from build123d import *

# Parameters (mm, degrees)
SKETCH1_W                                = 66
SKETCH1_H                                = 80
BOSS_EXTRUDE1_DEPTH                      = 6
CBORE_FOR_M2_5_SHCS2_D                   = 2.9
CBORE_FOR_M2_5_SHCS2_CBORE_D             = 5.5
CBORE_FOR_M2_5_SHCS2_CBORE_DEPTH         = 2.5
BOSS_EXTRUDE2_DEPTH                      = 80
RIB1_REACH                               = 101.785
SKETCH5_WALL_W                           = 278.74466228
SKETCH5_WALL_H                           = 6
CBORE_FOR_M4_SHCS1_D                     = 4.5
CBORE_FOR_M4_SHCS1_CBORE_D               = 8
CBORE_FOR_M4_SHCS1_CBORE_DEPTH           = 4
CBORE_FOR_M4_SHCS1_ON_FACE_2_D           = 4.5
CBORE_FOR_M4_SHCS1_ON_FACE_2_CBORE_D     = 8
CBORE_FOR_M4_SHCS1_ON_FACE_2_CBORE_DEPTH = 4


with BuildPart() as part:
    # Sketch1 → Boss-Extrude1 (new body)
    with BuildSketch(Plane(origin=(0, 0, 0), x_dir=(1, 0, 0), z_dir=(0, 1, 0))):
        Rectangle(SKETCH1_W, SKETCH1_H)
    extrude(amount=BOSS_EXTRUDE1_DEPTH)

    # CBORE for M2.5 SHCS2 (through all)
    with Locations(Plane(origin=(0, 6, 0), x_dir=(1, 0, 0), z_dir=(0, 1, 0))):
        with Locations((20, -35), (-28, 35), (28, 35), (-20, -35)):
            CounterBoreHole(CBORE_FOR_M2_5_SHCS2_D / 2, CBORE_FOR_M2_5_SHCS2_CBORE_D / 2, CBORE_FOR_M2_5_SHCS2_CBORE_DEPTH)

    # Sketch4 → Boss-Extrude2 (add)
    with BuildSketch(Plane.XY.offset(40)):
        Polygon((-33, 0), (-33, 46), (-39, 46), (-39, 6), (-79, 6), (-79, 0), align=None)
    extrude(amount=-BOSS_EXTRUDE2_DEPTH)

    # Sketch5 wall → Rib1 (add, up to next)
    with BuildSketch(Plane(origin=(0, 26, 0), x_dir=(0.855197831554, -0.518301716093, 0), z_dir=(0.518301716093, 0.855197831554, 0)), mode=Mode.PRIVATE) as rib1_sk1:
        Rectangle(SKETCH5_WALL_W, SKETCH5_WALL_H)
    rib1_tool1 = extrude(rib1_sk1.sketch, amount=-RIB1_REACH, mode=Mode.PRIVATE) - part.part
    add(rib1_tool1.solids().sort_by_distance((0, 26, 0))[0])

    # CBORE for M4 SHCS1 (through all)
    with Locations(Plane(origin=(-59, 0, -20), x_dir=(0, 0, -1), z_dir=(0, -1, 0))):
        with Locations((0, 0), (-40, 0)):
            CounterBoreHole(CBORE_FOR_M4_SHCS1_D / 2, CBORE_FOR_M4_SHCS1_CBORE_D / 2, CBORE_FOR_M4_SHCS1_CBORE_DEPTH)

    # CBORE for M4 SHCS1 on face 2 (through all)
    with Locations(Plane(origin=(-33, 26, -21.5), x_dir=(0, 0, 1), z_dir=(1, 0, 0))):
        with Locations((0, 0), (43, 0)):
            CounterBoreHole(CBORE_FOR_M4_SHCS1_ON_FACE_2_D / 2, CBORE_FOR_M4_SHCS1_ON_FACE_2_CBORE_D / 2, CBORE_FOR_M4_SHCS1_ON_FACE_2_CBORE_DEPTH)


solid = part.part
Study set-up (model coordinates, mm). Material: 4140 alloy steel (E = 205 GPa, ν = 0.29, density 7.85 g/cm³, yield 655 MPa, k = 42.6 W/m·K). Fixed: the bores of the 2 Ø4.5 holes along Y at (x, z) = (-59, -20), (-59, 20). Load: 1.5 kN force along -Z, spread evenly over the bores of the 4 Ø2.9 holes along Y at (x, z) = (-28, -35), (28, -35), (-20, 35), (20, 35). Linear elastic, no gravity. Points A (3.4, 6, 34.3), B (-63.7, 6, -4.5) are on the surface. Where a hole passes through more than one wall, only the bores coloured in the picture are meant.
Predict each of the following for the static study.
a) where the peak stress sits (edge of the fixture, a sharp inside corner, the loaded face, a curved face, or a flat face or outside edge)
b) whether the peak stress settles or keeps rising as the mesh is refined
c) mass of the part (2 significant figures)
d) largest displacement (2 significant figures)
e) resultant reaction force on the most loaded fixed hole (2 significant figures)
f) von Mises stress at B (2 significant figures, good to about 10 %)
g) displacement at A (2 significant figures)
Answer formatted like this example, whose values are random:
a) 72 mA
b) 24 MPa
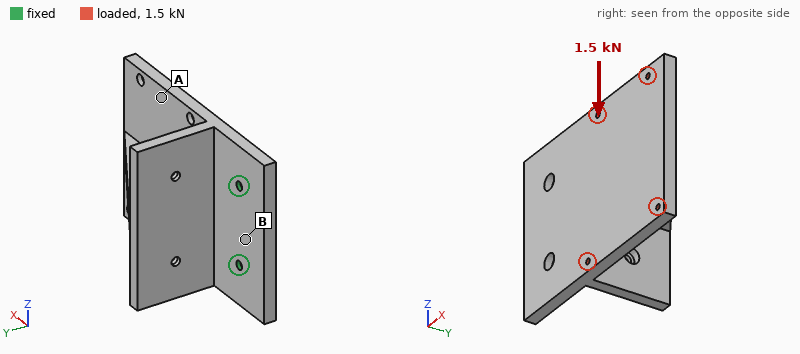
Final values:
a) edge of the fixture
b) keeps rising
c) 630 g
d) 19 µm
e) 2.3 kN
f) 12 MPa
g) 13 µm
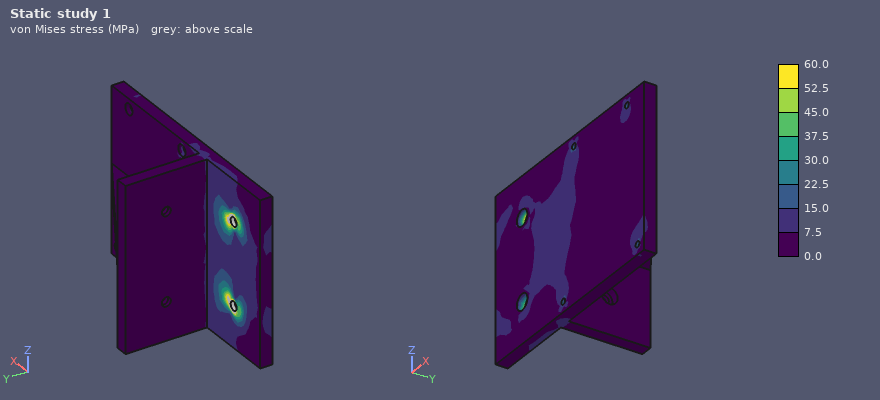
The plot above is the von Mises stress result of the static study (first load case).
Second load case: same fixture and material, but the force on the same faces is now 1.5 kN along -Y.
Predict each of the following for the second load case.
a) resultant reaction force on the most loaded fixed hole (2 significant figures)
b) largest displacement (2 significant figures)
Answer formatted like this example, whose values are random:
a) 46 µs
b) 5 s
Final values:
a) 790 N
b) 1.5 mm
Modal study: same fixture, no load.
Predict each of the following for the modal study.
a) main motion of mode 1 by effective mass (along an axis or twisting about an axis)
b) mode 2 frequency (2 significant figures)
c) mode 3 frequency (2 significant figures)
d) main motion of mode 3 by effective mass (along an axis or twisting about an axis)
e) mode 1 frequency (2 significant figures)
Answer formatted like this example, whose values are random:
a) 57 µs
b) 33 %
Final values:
a) along Y
b) 1500 Hz
c) 2800 Hz
d) along Z
e) 330 Hz
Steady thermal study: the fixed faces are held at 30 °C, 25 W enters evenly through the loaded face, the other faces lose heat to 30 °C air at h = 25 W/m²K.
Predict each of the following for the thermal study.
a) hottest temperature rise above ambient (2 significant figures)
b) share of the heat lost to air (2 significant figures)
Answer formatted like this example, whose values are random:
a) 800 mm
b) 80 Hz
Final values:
a) 60 K
b) 65 %
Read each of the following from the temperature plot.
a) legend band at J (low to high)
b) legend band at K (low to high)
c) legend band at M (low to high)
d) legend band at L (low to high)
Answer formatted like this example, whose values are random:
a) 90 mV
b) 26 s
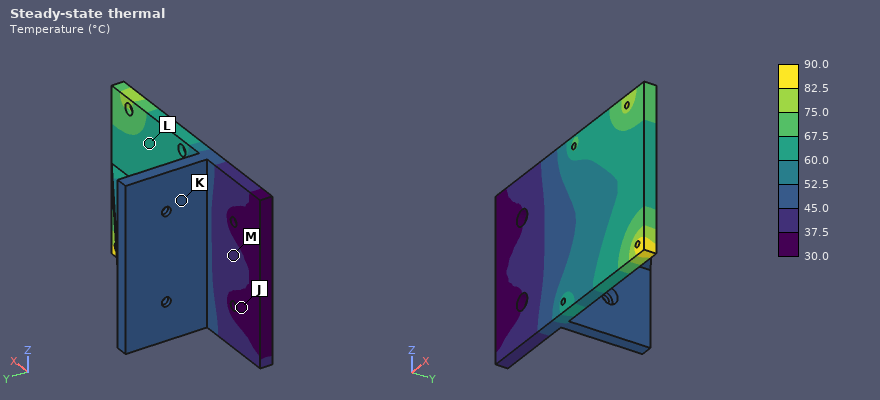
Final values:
a) 30.0 to 37.5 °C
b) 45.0 to 52.5 °C
c) 37.5 to 45.0 °C
d) 60.0 to 67.5 °C
